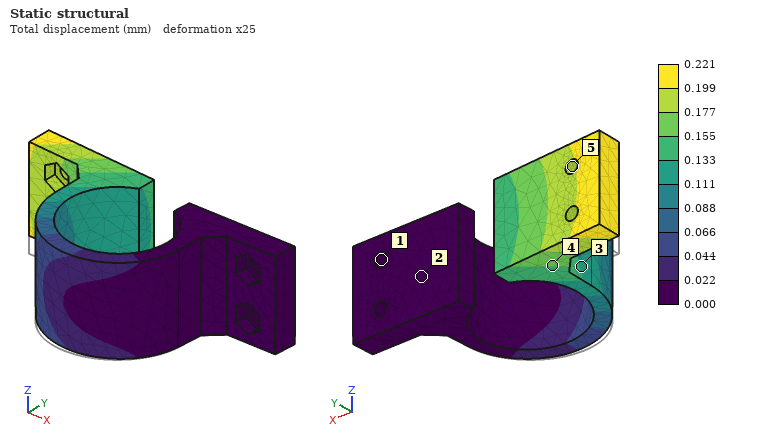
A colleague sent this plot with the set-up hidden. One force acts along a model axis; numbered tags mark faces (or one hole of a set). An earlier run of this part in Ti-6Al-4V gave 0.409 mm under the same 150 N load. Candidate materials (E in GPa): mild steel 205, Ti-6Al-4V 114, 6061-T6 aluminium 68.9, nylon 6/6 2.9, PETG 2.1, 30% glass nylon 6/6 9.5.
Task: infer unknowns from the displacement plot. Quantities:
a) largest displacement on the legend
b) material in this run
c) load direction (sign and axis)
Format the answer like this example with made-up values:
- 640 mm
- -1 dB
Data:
- 0.221 mm
- mild steel
- +Z
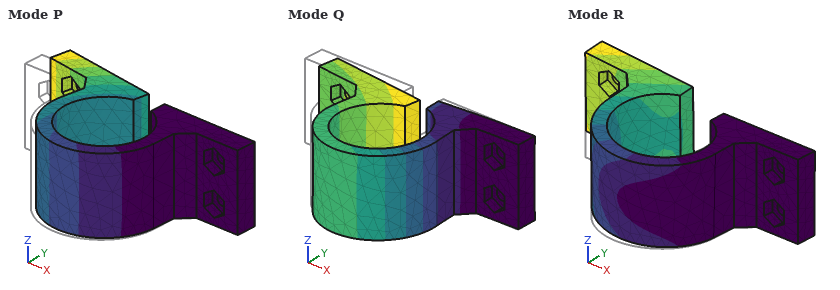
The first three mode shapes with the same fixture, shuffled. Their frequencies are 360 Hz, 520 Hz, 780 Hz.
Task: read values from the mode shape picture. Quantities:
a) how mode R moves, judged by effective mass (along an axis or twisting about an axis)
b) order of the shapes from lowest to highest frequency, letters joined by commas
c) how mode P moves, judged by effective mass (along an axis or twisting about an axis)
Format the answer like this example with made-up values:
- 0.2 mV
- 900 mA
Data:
- along Z
- P, R, Q
- along Y
